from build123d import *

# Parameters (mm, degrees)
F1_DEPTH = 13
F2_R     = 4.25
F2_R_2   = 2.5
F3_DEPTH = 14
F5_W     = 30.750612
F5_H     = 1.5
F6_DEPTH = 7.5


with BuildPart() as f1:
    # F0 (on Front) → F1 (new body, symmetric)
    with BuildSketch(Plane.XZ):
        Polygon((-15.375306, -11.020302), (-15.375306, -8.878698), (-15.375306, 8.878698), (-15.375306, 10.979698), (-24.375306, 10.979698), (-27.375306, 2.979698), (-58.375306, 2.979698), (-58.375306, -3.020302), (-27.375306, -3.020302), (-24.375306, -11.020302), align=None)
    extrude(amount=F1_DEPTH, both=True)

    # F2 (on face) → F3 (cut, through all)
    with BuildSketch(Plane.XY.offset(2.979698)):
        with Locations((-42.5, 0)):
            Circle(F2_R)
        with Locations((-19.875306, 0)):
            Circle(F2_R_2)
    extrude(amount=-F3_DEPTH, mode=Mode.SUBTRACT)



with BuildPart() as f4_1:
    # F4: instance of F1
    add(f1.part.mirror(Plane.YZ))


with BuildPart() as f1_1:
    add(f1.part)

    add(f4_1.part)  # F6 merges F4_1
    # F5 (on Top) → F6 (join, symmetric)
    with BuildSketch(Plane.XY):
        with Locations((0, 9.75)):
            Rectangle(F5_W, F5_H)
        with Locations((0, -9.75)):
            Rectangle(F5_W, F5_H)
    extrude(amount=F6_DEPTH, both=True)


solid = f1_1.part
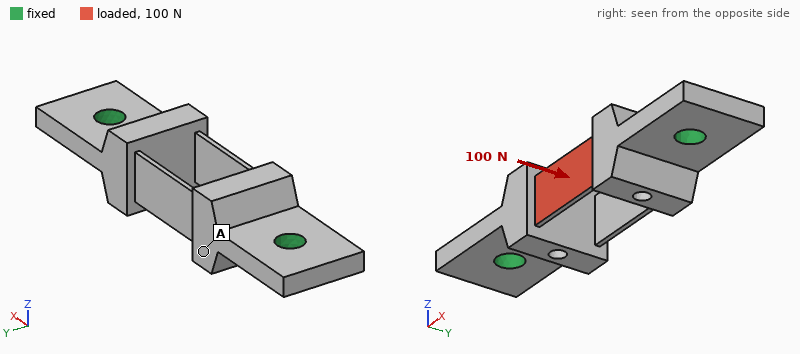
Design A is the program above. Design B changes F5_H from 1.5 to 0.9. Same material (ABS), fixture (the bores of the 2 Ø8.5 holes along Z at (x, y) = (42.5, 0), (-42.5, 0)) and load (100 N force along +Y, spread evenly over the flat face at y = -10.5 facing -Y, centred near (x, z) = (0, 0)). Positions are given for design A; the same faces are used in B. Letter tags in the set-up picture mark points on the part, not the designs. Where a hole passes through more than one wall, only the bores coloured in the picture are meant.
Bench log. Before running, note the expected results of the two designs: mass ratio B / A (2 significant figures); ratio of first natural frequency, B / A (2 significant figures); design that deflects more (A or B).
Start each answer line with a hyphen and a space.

- 0.98
- 0.94
- B
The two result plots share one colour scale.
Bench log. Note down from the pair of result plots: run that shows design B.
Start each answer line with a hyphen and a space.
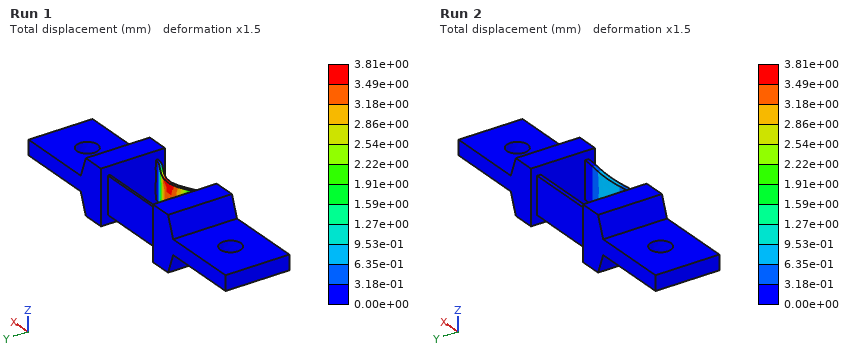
- Run 1
